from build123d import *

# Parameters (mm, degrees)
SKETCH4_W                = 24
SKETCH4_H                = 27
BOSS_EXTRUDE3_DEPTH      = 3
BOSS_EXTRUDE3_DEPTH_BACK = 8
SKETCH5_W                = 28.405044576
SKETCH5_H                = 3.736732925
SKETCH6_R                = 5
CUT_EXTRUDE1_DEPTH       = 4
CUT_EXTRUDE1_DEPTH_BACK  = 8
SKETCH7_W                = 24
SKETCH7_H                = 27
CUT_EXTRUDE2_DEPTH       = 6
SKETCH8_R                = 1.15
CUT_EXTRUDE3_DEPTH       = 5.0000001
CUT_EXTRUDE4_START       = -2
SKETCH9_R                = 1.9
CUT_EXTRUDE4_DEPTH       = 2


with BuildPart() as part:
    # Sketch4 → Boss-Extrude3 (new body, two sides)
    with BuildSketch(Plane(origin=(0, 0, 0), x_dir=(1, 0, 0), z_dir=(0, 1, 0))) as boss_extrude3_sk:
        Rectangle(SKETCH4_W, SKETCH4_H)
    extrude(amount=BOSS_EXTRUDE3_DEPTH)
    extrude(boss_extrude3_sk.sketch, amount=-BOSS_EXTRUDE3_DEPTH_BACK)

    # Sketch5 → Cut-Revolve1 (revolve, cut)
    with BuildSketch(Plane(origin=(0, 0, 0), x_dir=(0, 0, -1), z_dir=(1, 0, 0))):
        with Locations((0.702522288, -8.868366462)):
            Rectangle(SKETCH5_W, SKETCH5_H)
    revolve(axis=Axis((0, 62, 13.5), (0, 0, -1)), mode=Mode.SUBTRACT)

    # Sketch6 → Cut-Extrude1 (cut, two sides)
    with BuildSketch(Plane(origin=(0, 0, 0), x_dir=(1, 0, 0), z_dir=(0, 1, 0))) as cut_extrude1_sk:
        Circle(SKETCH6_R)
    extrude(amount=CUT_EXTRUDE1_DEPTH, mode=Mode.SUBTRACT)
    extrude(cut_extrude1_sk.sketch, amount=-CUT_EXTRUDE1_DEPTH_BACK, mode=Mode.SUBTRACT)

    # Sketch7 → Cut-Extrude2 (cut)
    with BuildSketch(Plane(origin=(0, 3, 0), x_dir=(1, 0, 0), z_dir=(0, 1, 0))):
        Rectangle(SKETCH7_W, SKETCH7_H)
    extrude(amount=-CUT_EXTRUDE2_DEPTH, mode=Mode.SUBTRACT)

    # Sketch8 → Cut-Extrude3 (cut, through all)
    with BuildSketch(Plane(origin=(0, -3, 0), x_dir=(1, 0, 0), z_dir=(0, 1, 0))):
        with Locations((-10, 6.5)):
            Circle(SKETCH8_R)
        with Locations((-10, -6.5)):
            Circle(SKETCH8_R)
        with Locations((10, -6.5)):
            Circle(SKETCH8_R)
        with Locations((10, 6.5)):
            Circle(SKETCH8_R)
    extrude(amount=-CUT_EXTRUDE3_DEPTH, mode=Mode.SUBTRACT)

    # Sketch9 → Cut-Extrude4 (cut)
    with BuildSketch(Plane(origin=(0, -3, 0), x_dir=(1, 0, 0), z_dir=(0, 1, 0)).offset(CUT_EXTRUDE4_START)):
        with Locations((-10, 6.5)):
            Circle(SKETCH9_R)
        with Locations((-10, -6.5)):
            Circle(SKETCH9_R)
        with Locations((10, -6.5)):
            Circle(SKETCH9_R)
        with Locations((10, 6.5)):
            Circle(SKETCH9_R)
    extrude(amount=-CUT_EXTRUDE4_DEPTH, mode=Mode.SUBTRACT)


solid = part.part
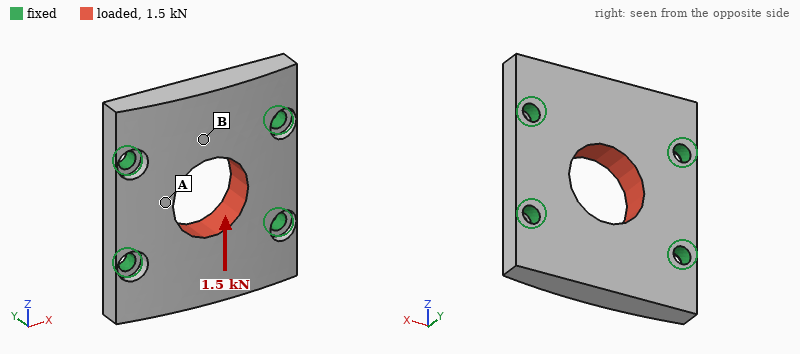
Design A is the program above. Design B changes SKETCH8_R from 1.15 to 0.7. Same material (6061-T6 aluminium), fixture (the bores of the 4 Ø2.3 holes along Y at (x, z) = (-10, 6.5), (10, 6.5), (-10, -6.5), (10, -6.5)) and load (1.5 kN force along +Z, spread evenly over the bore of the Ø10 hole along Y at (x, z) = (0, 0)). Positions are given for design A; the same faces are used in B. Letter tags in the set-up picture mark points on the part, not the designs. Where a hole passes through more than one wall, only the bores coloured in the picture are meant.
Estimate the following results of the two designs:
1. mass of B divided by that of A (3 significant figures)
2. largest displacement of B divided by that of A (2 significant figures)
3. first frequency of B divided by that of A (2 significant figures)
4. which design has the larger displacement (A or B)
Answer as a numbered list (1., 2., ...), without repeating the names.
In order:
1. 1.01
2. 1.2
3. 0.87
4. B
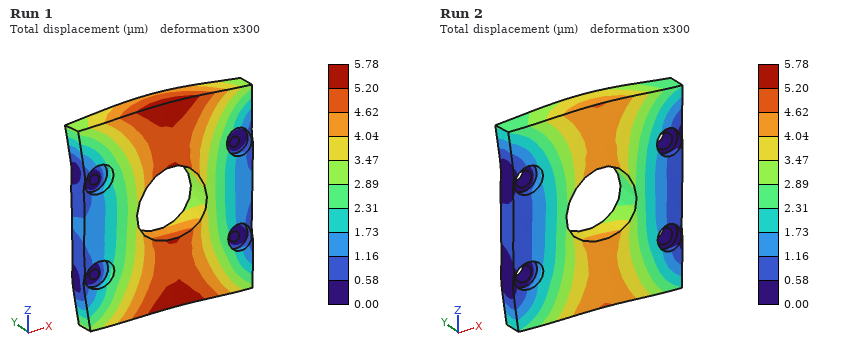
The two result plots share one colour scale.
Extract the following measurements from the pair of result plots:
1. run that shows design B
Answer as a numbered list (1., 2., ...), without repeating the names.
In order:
1. Run 1
